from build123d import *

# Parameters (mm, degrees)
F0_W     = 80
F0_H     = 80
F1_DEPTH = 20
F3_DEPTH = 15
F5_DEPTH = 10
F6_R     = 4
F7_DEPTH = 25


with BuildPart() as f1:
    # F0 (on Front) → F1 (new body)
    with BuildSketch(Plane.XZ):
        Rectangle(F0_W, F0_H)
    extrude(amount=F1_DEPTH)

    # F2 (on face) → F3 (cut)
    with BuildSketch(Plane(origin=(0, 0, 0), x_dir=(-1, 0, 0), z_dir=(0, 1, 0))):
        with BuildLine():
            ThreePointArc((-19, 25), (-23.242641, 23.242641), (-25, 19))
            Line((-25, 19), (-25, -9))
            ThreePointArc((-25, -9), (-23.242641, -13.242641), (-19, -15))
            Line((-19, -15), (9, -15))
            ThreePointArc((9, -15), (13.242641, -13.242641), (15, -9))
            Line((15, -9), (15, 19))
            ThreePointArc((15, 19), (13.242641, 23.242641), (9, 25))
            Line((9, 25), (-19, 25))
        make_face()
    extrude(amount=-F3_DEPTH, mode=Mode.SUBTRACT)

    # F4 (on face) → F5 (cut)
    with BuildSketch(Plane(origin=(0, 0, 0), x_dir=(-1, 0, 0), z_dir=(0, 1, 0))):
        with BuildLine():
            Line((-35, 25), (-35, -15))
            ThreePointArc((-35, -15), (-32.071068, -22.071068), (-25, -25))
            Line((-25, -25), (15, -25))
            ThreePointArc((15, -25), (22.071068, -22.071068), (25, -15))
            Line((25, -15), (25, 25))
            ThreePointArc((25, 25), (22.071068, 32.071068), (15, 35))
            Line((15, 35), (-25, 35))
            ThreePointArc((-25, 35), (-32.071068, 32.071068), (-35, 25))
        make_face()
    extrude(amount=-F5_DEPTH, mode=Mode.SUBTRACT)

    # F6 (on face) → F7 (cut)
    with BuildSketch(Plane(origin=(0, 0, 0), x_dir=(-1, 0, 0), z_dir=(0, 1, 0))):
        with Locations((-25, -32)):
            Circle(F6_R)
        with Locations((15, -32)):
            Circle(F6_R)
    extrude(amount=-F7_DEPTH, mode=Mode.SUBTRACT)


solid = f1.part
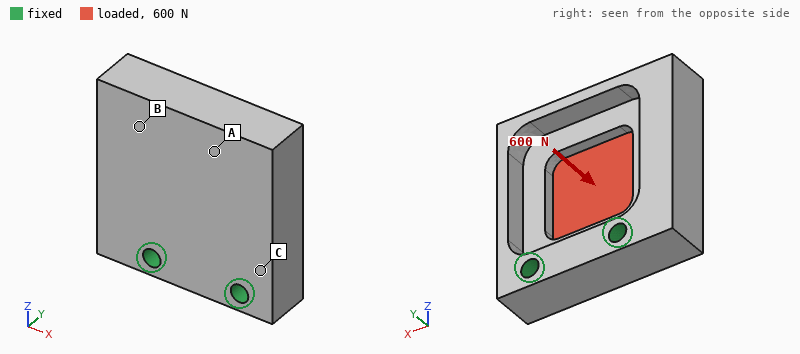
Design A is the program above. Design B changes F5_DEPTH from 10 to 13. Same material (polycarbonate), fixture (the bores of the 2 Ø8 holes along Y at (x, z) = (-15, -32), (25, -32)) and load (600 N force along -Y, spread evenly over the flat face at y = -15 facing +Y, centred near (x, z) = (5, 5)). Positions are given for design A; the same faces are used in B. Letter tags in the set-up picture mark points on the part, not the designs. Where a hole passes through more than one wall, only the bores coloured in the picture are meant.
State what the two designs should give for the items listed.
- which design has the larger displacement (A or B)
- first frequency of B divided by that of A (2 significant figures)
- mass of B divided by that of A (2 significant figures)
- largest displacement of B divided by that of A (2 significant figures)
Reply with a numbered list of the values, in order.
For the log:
1. B
2. 0.98
3. 0.93
4. 1.2
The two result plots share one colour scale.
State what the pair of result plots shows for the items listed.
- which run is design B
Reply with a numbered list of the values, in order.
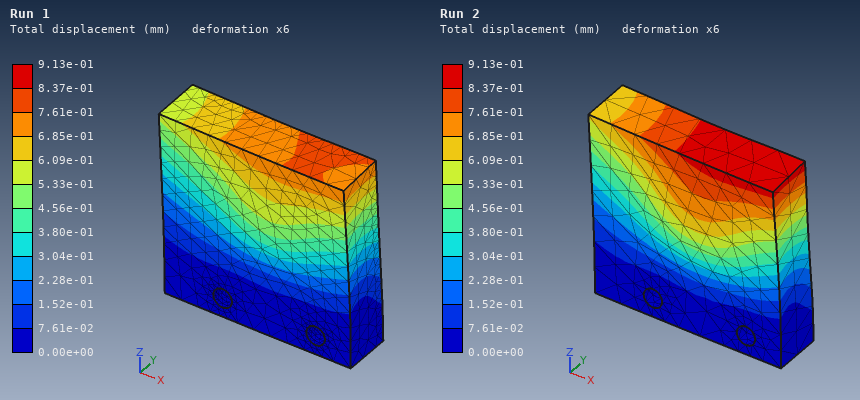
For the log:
1. Run 2
